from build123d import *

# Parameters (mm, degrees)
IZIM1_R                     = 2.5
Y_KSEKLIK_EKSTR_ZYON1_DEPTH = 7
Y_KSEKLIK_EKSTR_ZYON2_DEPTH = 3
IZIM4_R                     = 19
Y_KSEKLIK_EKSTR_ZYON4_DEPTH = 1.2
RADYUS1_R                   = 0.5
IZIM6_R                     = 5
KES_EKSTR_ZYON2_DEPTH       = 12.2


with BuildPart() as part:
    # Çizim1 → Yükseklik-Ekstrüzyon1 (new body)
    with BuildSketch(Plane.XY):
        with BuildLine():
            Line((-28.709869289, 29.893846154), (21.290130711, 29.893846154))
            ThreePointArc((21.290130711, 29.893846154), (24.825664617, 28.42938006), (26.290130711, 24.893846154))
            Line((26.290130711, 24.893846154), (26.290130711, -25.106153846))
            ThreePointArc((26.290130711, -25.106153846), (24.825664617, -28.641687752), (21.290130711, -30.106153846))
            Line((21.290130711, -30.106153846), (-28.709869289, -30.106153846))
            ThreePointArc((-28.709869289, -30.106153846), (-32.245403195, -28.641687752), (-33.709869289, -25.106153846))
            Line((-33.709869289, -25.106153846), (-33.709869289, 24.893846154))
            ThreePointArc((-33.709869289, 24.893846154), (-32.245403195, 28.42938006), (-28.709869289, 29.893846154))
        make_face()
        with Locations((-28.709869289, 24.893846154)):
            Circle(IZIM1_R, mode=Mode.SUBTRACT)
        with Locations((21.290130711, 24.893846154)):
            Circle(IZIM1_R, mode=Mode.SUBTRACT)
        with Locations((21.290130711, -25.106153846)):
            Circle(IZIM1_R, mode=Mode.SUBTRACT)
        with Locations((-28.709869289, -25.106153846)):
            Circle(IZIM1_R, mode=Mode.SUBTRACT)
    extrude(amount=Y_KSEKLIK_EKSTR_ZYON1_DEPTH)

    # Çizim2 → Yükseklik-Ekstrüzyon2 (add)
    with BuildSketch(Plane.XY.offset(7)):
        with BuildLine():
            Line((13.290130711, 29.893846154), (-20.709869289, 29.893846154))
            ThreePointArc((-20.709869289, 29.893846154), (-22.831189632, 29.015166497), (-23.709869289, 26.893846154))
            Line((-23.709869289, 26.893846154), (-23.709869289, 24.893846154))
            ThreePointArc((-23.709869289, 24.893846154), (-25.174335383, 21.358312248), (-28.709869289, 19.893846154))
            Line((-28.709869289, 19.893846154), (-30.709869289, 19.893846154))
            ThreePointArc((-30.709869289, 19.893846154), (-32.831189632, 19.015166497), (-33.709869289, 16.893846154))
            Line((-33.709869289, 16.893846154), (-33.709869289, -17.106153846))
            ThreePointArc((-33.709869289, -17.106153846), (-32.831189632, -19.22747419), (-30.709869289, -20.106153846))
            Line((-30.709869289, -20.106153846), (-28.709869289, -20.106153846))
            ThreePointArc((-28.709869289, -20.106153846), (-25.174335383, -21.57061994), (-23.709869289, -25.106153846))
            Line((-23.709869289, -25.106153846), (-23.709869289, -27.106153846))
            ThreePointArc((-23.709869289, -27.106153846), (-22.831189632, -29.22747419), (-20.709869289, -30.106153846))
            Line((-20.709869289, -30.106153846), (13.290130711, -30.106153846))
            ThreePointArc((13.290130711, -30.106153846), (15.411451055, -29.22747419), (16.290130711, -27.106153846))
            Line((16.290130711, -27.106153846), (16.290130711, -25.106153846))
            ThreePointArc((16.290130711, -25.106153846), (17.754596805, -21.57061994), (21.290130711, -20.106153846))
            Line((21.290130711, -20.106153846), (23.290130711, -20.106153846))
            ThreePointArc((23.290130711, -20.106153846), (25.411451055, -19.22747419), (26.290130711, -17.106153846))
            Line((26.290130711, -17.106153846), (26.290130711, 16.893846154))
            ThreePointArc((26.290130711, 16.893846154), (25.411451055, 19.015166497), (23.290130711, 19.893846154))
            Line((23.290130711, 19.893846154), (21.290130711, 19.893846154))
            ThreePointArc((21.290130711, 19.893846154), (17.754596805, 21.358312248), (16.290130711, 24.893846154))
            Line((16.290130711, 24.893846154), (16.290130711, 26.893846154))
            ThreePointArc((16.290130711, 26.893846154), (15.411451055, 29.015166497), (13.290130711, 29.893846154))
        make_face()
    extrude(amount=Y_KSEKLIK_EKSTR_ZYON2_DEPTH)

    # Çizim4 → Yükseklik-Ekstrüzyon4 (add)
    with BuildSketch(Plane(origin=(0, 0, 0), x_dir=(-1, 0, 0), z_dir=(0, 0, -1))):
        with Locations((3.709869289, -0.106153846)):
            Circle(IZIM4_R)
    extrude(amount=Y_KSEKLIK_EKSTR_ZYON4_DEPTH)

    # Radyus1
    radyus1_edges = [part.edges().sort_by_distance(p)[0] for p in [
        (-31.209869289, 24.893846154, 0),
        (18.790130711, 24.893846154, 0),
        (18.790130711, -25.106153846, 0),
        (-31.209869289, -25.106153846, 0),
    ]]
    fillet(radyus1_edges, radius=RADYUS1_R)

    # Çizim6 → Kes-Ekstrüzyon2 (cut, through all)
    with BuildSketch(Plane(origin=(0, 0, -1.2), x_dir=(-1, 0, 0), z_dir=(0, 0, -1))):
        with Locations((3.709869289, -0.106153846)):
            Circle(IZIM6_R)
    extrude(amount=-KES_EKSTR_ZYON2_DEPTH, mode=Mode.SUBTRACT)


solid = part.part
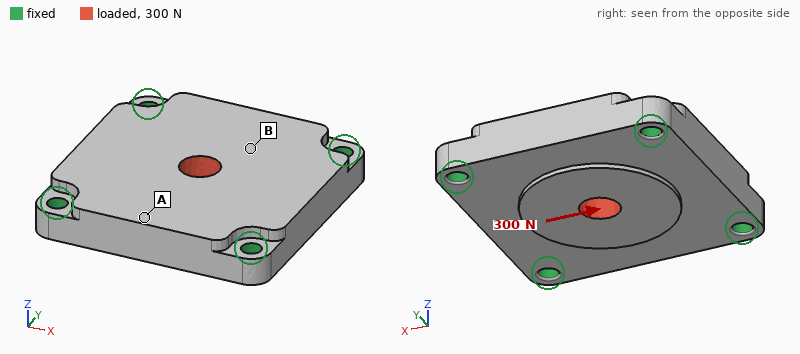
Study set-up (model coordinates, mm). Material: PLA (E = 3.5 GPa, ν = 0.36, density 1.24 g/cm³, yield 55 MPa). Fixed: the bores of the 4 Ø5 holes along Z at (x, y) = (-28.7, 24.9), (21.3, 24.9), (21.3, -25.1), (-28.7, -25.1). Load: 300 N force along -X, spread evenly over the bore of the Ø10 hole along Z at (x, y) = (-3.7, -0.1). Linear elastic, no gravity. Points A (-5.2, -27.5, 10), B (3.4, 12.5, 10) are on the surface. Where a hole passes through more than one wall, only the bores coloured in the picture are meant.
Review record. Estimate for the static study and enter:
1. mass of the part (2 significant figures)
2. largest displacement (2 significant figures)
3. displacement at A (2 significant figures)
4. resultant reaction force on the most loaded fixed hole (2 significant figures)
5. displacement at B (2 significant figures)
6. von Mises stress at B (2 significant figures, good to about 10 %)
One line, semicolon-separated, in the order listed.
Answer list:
43 g; 7.8 µm; 1.9 µm; 83 N; 4.2 µm; 0.48 MPa
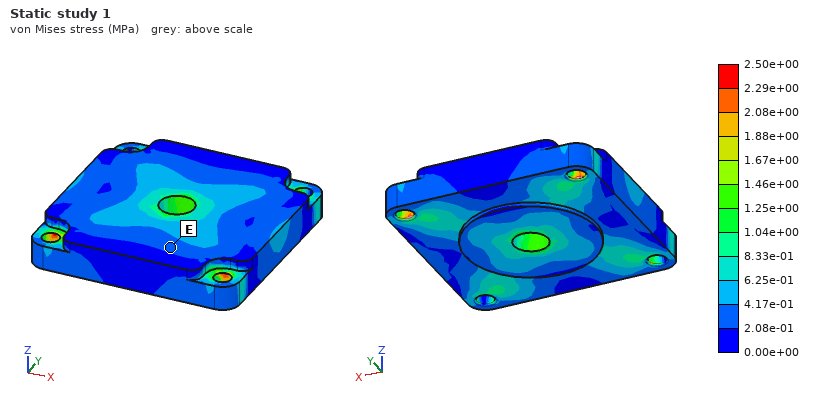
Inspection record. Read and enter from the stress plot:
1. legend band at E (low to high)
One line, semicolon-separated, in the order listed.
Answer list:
2.08e-01 to 4.17e-01 MPa
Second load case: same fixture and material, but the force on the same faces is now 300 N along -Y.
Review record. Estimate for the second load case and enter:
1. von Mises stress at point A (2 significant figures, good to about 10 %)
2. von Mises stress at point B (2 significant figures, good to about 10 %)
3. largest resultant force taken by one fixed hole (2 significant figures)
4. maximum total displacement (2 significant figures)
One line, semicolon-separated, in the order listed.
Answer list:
0.35 MPa; 0.49 MPa; 83 N; 7.8 µm
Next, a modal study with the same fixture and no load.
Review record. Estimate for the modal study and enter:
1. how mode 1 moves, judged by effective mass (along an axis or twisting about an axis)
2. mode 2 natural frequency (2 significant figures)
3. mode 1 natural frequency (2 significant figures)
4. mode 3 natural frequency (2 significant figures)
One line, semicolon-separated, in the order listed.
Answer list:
along Z; 5400 Hz; 3400 Hz; 5400 Hz
